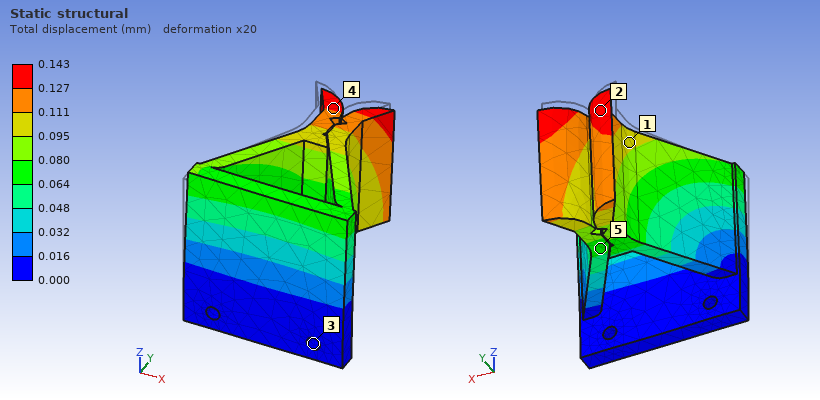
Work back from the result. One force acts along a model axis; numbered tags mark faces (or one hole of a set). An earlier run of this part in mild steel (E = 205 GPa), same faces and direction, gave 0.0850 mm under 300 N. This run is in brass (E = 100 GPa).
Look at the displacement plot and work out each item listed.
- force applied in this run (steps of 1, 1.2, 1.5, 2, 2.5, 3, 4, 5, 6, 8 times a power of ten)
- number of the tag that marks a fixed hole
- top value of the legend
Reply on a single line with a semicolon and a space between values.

250 N; 3; 0.143 mm
